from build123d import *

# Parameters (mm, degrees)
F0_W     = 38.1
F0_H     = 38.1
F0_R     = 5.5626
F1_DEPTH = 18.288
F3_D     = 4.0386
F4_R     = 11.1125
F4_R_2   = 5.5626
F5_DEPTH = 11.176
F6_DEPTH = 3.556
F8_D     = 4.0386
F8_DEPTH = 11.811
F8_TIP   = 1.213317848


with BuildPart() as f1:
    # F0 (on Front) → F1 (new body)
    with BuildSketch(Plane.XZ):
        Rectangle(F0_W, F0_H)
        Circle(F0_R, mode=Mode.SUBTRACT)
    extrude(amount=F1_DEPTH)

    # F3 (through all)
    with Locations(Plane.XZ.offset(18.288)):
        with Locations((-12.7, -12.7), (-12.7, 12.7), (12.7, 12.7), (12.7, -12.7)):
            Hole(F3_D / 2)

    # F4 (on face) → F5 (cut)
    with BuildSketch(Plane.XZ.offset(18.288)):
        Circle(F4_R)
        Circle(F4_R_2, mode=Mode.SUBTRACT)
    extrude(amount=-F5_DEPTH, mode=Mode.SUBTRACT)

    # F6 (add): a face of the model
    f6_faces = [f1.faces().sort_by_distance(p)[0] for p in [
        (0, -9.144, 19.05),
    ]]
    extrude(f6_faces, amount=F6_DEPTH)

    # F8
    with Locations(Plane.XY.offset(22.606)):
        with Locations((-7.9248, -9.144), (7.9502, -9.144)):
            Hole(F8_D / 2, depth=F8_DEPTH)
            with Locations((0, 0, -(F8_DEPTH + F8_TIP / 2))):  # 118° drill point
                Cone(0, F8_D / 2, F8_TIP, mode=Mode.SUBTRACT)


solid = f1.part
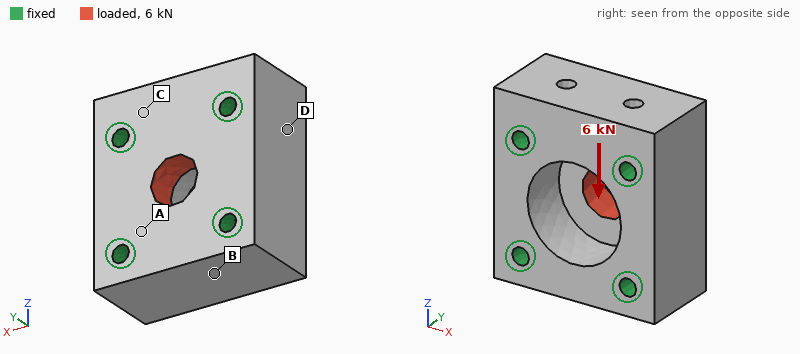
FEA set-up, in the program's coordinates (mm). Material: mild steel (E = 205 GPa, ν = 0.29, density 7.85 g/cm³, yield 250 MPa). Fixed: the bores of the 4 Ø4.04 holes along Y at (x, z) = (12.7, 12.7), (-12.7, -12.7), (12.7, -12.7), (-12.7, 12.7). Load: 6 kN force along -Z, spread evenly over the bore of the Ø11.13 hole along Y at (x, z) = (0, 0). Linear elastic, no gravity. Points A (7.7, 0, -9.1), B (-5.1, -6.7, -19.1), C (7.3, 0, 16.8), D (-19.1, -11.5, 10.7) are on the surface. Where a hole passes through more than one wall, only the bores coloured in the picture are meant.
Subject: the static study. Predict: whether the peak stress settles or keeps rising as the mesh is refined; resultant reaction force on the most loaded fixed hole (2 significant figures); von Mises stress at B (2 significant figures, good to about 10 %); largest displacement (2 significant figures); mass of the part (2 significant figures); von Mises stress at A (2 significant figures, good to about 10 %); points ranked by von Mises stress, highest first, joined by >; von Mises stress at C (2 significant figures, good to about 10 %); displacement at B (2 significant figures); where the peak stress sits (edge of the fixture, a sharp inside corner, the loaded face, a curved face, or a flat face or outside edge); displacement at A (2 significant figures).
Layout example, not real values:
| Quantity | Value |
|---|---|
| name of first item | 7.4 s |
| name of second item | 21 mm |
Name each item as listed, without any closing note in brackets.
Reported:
| Quantity | Value |
|---|---|
| whether the peak stress settles or keeps rising as the mesh is refined | keeps rising |
| resultant reaction force on the most loaded fixed hole | 1.6 kN |
| von Mises stress at B | 7.3 MPa |
| largest displacement | 1.8 µm |
| mass of the part | 180 g |
| von Mises stress at A | 23 MPa |
| points ranked by von Mises stress, highest first, joined by > | A > C > B > D |
| von Mises stress at C | 13 MPa |
| displacement at B | 0.64 µm |
| where the peak stress sits | edge of the fixture |
| displacement at A | 0.70 µm |
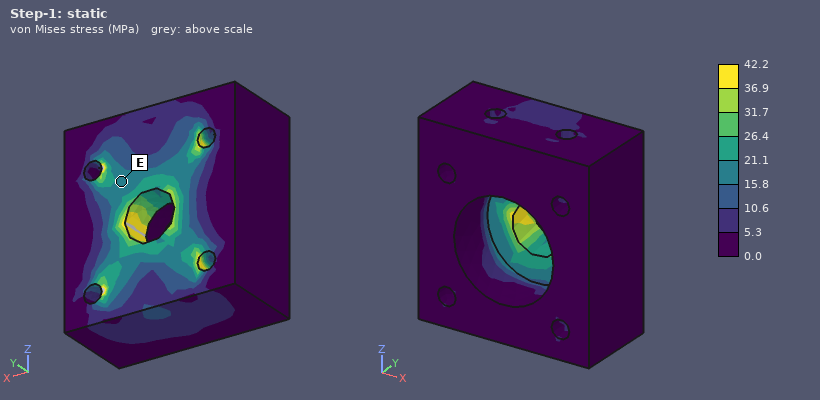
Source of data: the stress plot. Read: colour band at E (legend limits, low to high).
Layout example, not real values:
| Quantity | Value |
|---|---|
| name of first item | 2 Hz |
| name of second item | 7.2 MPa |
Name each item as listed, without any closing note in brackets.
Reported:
| Quantity | Value |
|---|---|
| colour band at E | 15.8 to 21.1 MPa |
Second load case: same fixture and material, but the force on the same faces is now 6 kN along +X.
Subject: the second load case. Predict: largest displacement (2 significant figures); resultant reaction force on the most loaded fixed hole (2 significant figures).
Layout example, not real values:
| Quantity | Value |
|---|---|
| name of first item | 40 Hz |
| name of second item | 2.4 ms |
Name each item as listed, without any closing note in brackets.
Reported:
| Quantity | Value |
|---|---|
| largest displacement | 1.9 µm |
| resultant reaction force on the most loaded fixed hole | 1.6 kN |
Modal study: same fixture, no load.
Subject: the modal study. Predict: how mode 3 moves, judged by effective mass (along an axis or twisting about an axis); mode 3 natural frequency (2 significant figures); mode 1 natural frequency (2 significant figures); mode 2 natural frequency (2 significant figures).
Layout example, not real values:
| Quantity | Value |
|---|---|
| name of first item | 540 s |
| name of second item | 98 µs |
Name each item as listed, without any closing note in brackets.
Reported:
| Quantity | Value |
|---|---|
| how mode 3 moves, judged by effective mass | along Y |
| mode 3 natural frequency | 53 kHz |
| mode 1 natural frequency | 45 kHz |
| mode 2 natural frequency | 46 kHz |
